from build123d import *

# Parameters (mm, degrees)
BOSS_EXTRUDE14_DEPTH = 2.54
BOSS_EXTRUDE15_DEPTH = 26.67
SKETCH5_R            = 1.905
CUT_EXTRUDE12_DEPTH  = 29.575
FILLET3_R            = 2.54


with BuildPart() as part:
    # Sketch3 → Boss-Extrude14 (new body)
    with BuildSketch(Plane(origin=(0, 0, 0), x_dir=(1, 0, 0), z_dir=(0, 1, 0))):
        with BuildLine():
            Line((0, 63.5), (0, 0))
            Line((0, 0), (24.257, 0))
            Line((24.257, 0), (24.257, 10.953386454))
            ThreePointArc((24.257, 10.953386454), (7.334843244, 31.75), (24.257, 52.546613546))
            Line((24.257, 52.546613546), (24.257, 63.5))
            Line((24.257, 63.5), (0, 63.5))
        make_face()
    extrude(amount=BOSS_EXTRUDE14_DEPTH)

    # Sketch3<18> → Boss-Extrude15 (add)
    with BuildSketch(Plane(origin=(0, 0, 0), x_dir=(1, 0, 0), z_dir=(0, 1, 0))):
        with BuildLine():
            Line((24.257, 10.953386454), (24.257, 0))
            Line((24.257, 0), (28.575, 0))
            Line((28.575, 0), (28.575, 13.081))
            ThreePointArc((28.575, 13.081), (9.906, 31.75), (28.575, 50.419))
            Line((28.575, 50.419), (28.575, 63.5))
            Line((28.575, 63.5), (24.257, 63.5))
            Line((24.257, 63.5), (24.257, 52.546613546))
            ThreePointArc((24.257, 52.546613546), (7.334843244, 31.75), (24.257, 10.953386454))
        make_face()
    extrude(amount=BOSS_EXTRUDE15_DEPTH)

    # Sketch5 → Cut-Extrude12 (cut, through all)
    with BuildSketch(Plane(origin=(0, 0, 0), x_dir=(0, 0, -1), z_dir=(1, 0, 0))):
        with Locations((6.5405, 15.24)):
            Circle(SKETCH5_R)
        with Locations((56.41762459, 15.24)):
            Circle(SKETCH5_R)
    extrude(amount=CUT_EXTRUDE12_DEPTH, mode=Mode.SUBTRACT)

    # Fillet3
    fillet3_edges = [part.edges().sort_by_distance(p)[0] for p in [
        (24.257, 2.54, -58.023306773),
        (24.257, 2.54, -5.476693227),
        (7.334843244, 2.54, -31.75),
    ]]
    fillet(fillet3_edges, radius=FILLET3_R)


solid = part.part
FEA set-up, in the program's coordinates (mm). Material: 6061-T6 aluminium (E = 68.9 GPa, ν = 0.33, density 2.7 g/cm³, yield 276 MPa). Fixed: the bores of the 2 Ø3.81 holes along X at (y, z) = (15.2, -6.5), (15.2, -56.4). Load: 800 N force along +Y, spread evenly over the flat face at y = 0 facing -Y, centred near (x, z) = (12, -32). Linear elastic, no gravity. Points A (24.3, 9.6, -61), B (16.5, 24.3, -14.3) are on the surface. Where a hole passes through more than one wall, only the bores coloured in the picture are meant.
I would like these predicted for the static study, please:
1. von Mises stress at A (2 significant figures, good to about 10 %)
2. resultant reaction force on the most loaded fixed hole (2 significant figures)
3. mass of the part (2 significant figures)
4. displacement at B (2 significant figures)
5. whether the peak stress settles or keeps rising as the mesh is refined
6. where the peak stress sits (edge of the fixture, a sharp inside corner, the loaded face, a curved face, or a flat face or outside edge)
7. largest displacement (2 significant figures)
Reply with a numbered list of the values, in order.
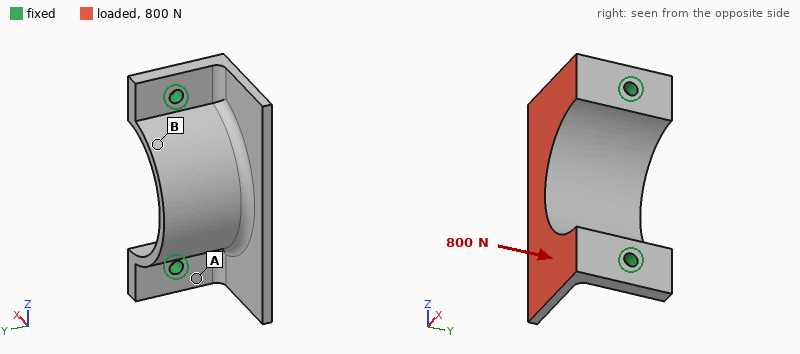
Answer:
1. 42 MPa
2. 410 N
3. 25 g
4. 0.034 mm
5. keeps rising
6. edge of the fixture
7. 0.17 mm
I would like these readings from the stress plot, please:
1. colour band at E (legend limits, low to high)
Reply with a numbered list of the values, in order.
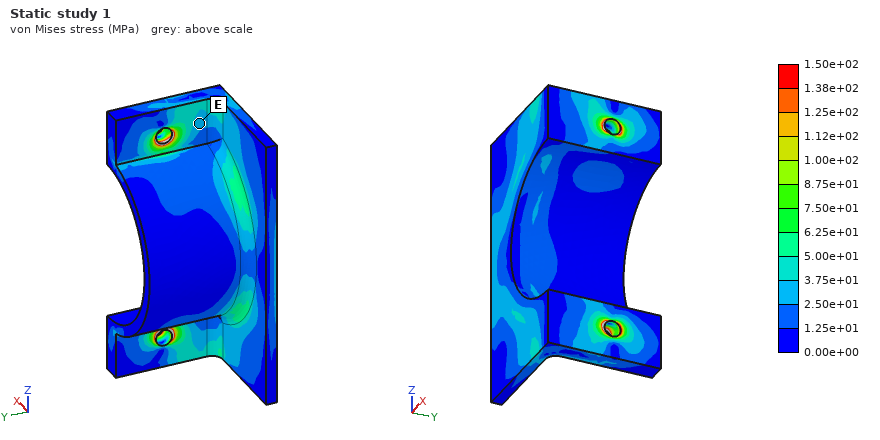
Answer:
1. 2.50e+01 to 3.75e+01 MPa
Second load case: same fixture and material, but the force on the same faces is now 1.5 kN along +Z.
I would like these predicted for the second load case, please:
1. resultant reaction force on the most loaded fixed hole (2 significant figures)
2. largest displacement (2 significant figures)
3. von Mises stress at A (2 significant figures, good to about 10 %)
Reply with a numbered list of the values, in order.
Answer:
1. 930 N
2. 50 µm
3. 27 MPa
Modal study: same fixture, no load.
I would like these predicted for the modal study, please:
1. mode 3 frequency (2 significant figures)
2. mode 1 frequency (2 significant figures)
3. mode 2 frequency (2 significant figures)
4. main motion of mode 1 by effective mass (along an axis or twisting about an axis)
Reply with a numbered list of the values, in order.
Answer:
1. 7900 Hz
2. 4000 Hz
3. 5600 Hz
4. along Y
